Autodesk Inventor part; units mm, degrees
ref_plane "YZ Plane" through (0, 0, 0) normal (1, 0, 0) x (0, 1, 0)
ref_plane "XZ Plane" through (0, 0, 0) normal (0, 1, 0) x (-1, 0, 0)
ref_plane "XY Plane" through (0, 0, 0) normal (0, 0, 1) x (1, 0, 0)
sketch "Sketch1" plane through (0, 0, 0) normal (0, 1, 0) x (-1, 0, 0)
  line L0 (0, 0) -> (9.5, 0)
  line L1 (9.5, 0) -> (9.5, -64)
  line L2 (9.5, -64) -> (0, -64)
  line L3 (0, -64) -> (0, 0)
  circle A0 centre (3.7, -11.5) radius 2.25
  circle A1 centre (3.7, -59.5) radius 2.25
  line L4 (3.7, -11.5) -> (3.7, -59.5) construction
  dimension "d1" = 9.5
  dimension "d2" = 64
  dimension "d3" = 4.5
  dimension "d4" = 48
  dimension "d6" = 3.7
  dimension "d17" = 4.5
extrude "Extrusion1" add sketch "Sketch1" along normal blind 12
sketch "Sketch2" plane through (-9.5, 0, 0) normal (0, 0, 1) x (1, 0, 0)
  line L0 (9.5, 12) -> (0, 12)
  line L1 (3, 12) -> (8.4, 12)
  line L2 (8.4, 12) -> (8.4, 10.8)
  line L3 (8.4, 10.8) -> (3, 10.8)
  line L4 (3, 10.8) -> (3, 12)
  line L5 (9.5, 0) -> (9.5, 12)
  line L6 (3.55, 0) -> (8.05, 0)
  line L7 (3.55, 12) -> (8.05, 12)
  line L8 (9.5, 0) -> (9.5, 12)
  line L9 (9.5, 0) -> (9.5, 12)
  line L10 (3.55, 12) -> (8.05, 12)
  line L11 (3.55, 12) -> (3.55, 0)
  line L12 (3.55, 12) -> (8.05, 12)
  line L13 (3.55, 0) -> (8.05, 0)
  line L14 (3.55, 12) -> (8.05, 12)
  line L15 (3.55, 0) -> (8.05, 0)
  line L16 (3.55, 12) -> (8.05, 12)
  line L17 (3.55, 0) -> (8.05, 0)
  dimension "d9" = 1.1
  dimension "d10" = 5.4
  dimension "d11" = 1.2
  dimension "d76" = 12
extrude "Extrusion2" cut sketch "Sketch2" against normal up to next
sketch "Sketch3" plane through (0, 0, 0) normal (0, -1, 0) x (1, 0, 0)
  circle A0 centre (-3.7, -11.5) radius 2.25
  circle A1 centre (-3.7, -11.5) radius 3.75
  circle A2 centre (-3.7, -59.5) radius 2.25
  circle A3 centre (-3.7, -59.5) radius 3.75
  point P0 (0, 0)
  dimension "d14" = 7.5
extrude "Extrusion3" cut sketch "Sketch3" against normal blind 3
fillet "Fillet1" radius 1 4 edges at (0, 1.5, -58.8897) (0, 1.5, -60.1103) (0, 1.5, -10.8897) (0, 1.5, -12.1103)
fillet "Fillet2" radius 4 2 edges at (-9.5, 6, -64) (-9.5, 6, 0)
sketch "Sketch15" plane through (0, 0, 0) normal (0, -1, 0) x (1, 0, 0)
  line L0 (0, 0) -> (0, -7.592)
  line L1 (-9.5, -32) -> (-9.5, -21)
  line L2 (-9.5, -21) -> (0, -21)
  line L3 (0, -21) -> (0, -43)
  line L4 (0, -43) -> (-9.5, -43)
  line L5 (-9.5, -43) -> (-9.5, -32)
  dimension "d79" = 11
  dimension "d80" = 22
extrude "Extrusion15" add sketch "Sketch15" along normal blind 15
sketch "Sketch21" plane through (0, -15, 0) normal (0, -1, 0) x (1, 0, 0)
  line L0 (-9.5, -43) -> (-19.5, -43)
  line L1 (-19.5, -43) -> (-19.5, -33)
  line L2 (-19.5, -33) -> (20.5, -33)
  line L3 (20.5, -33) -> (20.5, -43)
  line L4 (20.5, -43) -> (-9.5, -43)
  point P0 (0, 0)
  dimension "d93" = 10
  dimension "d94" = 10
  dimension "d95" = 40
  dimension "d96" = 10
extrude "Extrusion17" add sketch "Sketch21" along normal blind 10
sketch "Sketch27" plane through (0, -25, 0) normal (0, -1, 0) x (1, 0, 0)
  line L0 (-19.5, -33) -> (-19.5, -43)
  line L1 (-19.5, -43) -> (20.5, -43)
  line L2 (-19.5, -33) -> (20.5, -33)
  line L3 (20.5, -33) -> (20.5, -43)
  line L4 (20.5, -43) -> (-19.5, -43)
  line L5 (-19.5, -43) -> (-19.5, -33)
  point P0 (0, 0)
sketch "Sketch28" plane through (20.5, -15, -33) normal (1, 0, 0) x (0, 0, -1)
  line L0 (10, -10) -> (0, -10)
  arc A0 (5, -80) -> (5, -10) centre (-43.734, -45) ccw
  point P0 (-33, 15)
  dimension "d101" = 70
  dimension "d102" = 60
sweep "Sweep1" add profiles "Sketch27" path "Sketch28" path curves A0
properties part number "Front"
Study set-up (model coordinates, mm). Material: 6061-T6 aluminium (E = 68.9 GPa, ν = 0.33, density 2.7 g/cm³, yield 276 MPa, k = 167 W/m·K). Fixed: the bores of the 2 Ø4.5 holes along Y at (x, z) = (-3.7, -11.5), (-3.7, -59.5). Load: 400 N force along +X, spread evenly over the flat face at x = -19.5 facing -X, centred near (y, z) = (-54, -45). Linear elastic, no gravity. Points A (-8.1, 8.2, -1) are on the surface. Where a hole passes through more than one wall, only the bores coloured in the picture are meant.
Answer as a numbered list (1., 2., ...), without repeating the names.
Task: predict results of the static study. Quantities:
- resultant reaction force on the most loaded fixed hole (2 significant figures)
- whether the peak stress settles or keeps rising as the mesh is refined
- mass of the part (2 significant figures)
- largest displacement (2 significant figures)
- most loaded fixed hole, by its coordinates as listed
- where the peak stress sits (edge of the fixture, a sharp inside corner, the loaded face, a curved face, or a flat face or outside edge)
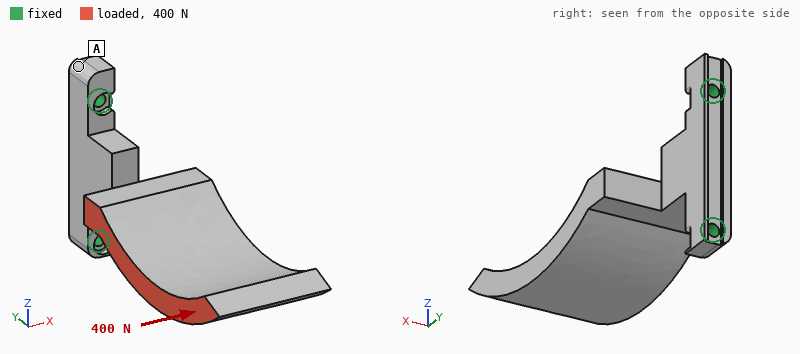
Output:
1. 280 N
2. keeps rising
3. 100 g
4. 1.1 mm
5. (-3.7, -59.5)
6. edge of the fixture
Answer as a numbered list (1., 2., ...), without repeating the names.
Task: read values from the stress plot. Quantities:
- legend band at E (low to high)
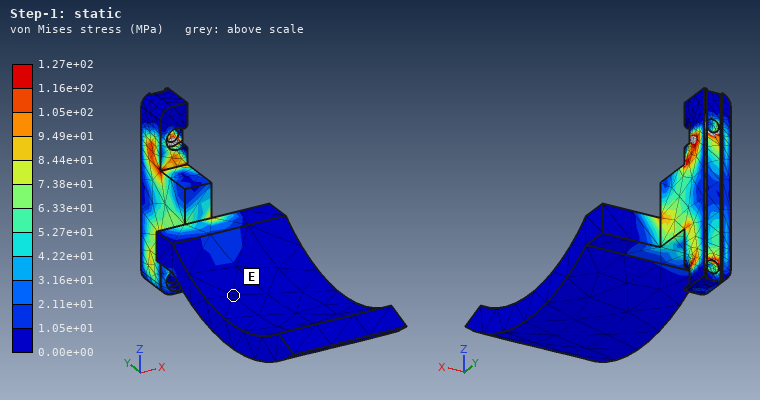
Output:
1. 0.00e+00 to 1.05e+01 MPa
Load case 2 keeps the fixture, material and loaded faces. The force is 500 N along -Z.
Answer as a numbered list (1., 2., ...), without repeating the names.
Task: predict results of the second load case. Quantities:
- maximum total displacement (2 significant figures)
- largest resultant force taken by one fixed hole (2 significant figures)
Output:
1. 0.65 mm
2. 850 N
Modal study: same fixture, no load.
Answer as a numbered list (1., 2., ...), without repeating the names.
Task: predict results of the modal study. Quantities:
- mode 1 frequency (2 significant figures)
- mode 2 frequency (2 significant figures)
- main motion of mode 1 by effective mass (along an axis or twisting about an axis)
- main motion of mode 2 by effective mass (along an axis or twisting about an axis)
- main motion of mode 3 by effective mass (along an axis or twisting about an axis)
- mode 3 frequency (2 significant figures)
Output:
1. 420 Hz
2. 650 Hz
3. along X
4. along Z
5. twisting about Y
6. 2100 Hz
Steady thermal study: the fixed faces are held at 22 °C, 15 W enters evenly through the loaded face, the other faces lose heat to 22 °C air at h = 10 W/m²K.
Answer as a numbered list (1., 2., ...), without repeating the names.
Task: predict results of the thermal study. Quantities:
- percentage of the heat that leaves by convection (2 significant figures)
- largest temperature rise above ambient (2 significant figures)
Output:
1. 14 %
2. 28 K
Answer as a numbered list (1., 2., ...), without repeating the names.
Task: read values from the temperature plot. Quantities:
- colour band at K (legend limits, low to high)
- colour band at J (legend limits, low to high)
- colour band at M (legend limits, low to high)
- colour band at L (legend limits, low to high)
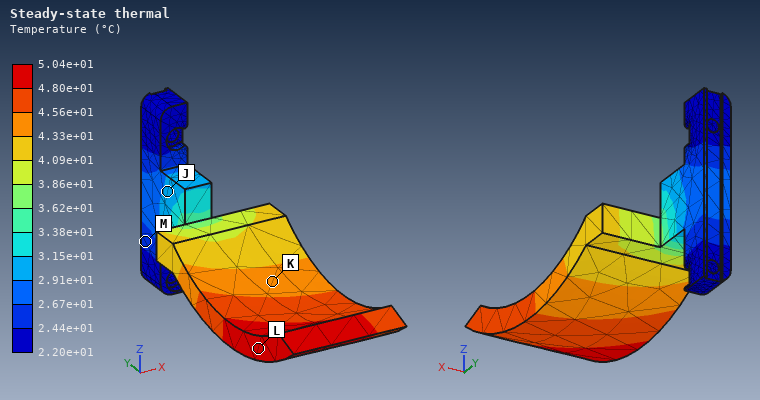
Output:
1. 4.33e+01 to 4.56e+01 °C
2. 2.91e+01 to 3.15e+01 °C
3. 2.44e+01 to 2.67e+01 °C
4. 4.80e+01 to 5.04e+01 °C
